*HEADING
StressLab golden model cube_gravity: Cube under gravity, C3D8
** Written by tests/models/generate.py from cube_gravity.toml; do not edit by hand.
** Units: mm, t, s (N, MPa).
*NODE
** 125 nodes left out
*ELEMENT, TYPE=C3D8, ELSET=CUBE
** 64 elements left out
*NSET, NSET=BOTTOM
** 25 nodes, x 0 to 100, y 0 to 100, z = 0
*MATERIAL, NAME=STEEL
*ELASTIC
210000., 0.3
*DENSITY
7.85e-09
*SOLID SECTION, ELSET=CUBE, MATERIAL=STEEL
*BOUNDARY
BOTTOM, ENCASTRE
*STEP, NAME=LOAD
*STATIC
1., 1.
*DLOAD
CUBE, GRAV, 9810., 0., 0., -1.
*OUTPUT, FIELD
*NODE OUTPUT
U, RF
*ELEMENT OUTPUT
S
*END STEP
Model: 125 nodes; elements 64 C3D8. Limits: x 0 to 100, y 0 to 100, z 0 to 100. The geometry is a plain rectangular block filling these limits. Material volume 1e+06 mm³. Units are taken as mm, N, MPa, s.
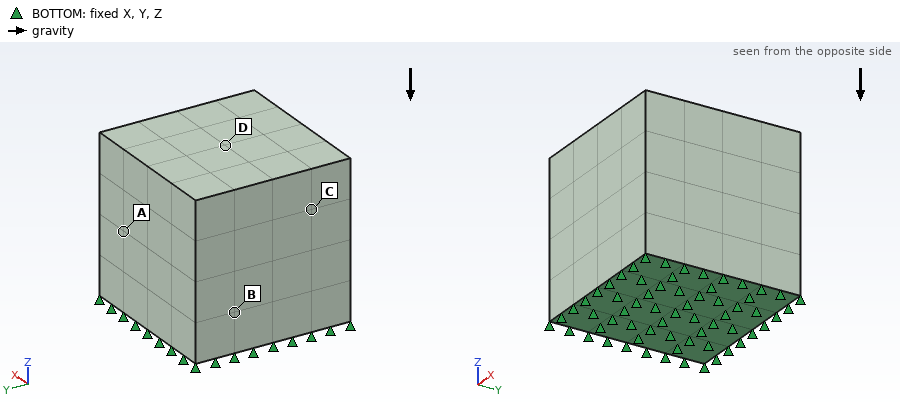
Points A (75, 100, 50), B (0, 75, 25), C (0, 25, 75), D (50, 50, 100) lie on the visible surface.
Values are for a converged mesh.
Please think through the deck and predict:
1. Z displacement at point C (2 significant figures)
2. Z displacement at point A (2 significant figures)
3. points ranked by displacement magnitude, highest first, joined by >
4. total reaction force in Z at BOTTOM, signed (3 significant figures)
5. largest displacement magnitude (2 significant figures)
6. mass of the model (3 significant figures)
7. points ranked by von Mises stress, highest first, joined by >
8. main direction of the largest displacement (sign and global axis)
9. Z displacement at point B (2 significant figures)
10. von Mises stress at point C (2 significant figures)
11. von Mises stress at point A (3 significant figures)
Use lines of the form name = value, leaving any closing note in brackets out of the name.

Z displacement at point C = -1.5e-06 mm
Z displacement at point A = -1.2e-06 mm
points ranked by displacement magnitude, highest first, joined by > = D > C > A > B
total reaction force in Z at BOTTOM, signed = 77.0 N
largest displacement magnitude = 1.8e-06 mm
mass of the model = 7.85 kg
points ranked by von Mises stress, highest first, joined by > = B > A > C > D
main direction of the largest displacement = -Z
Z displacement at point B = -7.3e-07 mm
von Mises stress at point C = 0.0019 MPa
von Mises stress at point A = 0.00345 MPa
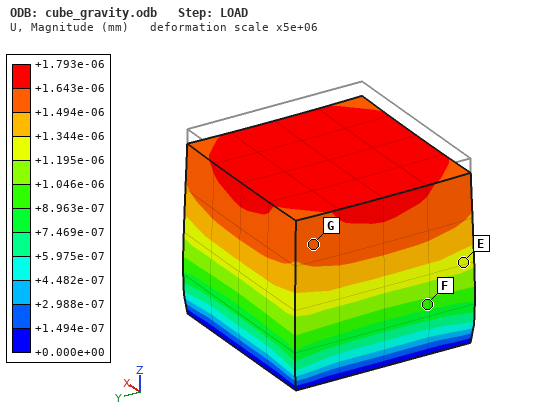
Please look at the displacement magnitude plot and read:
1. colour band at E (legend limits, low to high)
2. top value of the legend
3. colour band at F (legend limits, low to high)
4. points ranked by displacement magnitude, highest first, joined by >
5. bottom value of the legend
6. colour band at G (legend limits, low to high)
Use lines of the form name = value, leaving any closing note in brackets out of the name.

colour band at E = +1.195e-06 to +1.344e-06 mm
top value of the legend = +1.793e-06 mm
colour band at F = +8.963e-07 to +1.046e-06 mm
points ranked by displacement magnitude, highest first, joined by > = G > E > F
bottom value of the legend = +0.000e+00 mm
colour band at G = +1.494e-06 to +1.643e-06 mm
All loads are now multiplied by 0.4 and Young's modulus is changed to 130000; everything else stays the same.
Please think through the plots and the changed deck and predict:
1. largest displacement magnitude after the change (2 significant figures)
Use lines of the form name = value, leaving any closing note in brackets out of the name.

largest displacement magnitude after the change = 1.2e-06 mm
